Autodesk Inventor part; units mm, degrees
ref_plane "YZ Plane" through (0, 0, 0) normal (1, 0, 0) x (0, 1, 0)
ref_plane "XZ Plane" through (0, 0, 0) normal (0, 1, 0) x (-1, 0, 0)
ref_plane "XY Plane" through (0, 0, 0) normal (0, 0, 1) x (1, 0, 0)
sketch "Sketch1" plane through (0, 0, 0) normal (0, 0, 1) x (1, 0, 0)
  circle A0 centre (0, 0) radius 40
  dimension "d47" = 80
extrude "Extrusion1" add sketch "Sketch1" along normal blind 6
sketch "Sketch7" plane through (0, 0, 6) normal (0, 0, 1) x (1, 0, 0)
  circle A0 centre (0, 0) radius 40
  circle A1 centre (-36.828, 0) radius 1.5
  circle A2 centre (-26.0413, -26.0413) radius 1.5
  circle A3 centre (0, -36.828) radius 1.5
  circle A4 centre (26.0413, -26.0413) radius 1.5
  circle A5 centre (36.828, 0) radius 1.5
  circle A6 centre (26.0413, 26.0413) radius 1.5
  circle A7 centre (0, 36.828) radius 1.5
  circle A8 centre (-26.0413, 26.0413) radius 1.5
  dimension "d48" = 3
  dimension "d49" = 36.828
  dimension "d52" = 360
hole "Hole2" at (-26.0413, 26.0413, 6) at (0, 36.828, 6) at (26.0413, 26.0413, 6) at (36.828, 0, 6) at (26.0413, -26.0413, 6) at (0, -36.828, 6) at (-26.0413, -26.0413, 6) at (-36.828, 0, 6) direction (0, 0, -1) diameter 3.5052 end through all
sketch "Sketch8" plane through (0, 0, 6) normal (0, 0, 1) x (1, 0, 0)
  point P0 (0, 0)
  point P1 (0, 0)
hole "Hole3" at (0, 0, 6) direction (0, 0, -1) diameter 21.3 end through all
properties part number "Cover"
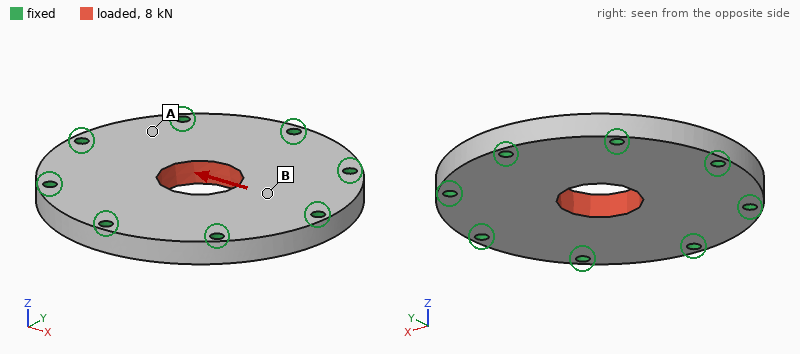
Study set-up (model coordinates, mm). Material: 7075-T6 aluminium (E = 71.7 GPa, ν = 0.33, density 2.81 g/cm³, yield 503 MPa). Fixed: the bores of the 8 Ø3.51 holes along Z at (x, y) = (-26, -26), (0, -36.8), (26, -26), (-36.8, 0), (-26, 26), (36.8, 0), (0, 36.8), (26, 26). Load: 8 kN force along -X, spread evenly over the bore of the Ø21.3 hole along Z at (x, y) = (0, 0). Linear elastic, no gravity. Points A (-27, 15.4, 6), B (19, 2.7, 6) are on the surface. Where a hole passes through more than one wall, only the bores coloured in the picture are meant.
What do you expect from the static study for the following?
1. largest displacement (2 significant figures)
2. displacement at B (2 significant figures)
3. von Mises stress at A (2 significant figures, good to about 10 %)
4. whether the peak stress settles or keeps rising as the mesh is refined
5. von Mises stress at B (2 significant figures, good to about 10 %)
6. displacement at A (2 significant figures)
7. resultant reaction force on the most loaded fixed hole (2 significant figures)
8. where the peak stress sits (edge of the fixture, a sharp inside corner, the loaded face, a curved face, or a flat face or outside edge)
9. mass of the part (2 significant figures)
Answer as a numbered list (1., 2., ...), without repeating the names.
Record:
1. 7.4 µm
2. 5.1 µm
3. 5.2 MPa
4. keeps rising
5. 18 MPa
6. 3.1 µm
7. 1.6 kN
8. edge of the fixture
9. 77 g
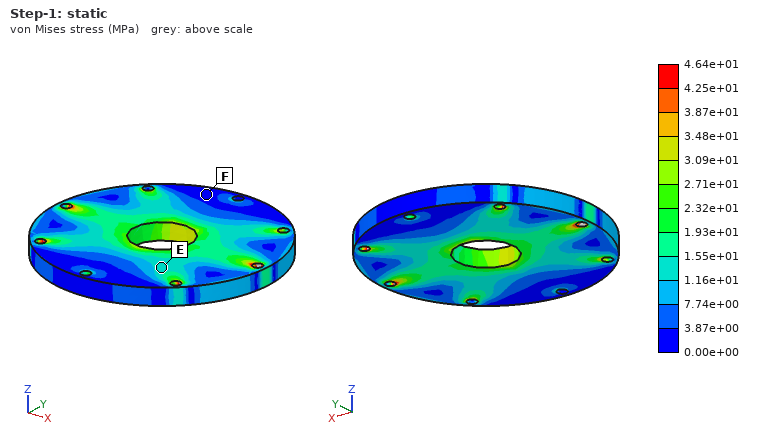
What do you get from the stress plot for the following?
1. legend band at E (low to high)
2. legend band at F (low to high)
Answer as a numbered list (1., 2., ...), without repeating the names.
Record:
1. 1.16e+01 to 1.55e+01 MPa
2. 0.00e+00 to 3.87e+00 MPa
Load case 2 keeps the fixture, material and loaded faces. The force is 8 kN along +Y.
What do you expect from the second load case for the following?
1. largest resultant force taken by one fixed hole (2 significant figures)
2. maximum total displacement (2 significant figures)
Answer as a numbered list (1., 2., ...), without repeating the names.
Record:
1. 1.6 kN
2. 7.4 µm
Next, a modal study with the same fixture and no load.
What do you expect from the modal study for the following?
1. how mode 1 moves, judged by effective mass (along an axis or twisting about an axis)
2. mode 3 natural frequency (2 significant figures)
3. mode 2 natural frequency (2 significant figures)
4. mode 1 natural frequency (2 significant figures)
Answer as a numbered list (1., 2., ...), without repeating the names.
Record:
1. along Z
2. 16 kHz
3. 16 kHz
4. 9200 Hz
